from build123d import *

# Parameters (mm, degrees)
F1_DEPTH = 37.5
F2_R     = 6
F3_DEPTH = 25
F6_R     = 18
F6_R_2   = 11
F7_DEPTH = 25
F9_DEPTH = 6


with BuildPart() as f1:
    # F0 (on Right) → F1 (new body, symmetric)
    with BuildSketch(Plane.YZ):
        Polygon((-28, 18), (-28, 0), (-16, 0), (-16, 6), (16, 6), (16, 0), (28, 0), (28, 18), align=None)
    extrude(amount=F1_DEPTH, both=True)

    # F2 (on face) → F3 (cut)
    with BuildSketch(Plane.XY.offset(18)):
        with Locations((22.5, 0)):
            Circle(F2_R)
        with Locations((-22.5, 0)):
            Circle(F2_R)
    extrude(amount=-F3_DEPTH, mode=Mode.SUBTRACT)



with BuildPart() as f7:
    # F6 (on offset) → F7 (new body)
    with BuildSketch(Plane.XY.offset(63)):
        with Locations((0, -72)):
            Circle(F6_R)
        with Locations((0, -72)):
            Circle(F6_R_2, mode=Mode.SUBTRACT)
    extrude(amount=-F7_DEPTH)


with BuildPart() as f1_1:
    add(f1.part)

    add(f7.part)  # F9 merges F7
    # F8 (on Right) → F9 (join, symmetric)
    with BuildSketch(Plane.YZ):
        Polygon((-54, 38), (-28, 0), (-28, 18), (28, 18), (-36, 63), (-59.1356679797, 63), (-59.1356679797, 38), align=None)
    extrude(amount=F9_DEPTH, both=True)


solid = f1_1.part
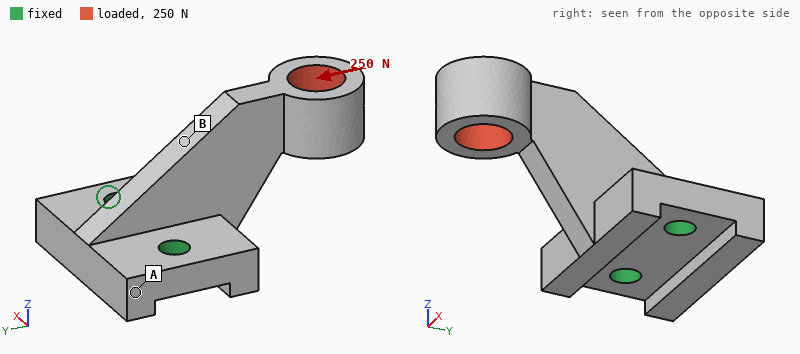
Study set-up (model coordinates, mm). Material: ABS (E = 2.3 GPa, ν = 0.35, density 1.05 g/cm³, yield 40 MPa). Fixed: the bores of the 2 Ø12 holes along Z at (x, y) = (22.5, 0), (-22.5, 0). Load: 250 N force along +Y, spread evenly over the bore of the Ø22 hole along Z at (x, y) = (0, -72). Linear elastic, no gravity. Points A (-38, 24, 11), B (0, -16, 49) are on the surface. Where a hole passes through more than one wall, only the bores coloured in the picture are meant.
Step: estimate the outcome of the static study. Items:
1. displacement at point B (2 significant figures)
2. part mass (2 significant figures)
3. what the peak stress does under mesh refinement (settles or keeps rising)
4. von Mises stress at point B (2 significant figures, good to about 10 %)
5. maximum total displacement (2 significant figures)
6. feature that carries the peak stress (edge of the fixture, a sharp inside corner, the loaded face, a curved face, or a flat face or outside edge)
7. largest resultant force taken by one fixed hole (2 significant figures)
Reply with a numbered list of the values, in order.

1. 0.14 mm
2. 110 g
3. keeps rising
4. 1.9 MPa
5. 0.42 mm
6. edge of the fixture
7. 130 N
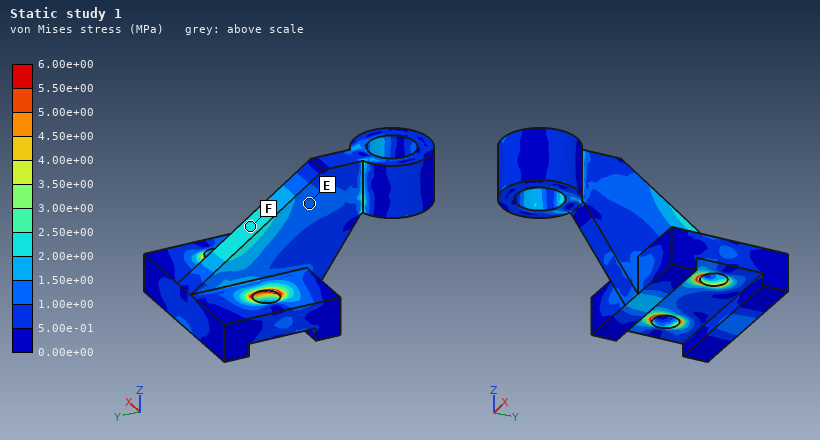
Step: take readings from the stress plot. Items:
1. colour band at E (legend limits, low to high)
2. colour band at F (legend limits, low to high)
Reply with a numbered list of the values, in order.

1. 1.00e+00 to 1.50e+00 MPa
2. 2.00e+00 to 2.50e+00 MPa
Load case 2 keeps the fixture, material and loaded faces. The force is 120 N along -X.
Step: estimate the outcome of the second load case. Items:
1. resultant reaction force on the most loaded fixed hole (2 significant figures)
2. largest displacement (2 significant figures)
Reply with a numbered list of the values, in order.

1. 210 N
2. 1.5 mm
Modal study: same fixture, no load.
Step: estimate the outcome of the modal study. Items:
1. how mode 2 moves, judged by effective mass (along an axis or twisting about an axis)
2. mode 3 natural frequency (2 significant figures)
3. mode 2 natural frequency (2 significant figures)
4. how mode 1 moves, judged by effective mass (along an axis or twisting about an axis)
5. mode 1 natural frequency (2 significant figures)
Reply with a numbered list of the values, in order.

1. along Z
2. 1100 Hz
3. 610 Hz
4. along X
5. 380 Hz
